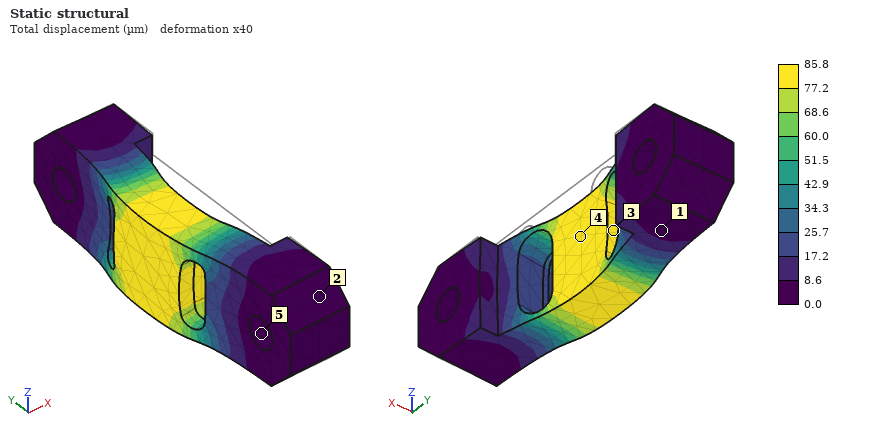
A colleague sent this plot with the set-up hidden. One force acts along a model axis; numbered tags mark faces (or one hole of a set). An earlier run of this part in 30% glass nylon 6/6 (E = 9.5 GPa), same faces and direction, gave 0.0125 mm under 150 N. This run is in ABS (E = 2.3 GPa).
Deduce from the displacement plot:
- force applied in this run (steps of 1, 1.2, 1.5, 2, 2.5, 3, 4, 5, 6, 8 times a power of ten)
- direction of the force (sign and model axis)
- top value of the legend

250 N
-X
85.8 µm
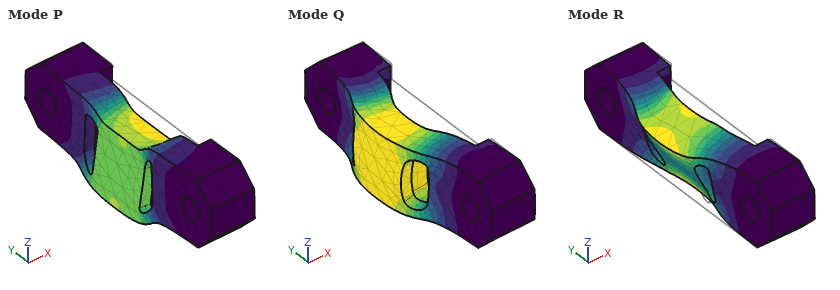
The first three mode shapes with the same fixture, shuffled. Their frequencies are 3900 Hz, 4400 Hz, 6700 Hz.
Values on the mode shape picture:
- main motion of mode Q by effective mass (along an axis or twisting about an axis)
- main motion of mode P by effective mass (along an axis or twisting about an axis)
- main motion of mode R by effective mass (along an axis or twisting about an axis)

along X
along Z
twisting about Y
